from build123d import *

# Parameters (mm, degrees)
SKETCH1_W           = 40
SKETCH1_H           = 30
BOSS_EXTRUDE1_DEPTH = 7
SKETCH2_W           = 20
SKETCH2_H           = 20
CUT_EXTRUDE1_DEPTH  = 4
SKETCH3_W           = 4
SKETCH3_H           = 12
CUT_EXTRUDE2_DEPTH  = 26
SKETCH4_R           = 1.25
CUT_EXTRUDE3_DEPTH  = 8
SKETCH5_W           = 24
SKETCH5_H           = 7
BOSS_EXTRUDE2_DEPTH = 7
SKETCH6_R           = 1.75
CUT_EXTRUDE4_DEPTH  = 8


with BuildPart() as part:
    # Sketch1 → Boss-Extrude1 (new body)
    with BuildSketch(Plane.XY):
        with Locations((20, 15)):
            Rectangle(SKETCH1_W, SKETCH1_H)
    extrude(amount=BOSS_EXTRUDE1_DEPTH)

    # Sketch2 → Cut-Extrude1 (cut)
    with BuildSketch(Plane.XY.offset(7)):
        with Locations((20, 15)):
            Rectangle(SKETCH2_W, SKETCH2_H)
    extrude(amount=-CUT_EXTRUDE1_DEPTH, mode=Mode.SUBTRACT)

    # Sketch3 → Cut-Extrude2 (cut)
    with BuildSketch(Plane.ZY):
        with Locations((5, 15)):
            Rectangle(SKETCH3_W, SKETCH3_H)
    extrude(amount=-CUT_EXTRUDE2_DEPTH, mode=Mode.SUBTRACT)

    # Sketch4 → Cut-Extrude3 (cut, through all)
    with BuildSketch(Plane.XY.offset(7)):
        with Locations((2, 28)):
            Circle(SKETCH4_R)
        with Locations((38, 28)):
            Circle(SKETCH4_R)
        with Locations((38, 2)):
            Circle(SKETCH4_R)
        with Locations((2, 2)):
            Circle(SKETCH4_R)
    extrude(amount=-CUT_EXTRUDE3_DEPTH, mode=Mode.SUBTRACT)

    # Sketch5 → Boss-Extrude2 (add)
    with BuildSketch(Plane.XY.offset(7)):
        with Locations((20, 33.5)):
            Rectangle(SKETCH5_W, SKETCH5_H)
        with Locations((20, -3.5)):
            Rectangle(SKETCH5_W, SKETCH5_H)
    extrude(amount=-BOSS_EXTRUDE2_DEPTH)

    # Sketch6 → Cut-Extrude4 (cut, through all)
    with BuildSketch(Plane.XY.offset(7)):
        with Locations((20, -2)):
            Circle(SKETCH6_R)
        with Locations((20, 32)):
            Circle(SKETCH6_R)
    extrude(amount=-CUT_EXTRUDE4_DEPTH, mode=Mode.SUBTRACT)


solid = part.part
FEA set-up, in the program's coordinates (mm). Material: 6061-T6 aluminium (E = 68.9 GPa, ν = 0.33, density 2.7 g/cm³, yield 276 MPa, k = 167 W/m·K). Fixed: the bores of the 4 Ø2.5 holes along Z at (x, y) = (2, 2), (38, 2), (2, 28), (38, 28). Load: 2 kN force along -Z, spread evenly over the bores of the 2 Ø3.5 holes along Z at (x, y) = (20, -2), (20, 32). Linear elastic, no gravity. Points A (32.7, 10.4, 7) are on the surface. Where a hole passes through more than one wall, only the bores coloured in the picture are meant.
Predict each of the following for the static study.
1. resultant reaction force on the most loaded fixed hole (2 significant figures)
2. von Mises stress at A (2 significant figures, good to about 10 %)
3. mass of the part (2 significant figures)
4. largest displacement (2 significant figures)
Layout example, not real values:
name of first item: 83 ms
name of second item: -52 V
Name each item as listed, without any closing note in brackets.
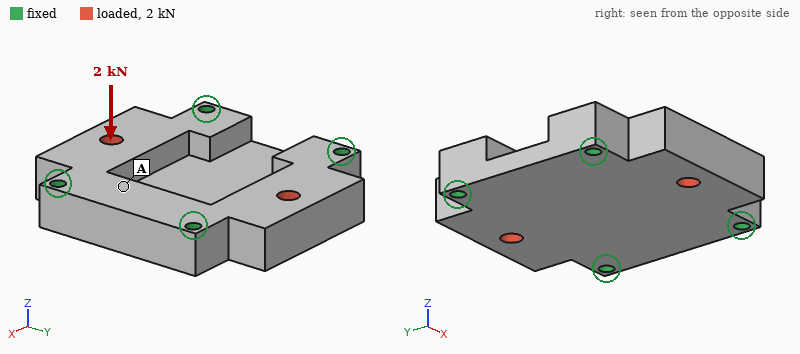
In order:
resultant reaction force on the most loaded fixed hole: 530 N
von Mises stress at A: 19 MPa
mass of the part: 23 g
largest displacement: 38 µm
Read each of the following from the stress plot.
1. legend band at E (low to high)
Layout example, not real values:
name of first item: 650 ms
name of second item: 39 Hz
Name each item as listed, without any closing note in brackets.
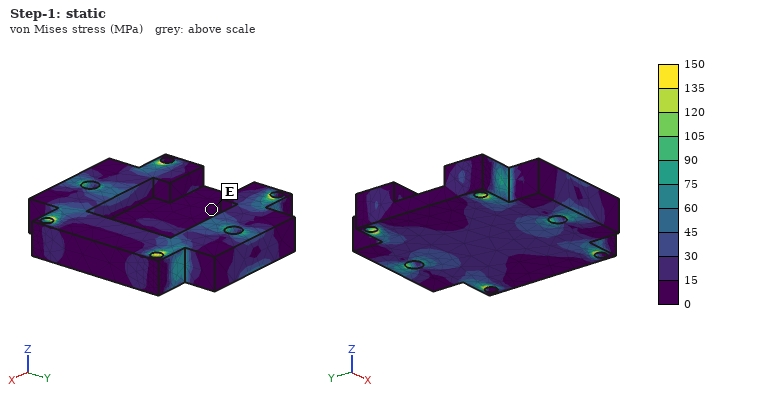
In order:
legend band at E: 0 to 15 MPa
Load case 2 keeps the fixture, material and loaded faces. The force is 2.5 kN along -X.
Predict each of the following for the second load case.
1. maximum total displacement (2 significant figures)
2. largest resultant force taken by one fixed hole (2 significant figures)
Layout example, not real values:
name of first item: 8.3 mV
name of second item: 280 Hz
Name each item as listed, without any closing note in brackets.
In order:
maximum total displacement: 4.8 µm
largest resultant force taken by one fixed hole: 630 N
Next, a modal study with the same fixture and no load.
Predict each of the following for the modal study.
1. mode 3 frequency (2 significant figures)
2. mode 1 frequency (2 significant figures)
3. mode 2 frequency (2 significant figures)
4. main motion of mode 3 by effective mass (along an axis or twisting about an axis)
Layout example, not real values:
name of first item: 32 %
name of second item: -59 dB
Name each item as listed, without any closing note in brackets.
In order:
mode 3 frequency: 21 kHz
mode 1 frequency: 15 kHz
mode 2 frequency: 15 kHz
main motion of mode 3 by effective mass: along Z
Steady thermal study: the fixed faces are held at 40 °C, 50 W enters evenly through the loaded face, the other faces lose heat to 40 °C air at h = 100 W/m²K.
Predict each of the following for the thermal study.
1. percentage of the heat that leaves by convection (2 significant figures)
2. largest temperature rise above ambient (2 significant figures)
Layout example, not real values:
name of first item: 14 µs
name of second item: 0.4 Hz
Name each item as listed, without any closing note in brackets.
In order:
percentage of the heat that leaves by convection: 8.0 %
largest temperature rise above ambient: 21 K
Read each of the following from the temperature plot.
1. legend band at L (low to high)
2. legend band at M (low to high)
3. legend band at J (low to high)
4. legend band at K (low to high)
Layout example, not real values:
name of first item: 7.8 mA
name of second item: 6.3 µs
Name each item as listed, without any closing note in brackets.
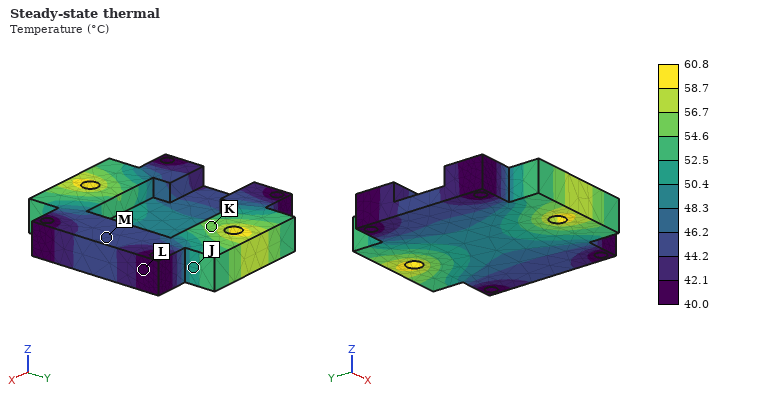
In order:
legend band at L: 40.0 to 42.1 °C
legend band at M: 44.2 to 46.2 °C
legend band at J: 50.4 to 52.5 °C
legend band at K: 54.6 to 56.7 °C
